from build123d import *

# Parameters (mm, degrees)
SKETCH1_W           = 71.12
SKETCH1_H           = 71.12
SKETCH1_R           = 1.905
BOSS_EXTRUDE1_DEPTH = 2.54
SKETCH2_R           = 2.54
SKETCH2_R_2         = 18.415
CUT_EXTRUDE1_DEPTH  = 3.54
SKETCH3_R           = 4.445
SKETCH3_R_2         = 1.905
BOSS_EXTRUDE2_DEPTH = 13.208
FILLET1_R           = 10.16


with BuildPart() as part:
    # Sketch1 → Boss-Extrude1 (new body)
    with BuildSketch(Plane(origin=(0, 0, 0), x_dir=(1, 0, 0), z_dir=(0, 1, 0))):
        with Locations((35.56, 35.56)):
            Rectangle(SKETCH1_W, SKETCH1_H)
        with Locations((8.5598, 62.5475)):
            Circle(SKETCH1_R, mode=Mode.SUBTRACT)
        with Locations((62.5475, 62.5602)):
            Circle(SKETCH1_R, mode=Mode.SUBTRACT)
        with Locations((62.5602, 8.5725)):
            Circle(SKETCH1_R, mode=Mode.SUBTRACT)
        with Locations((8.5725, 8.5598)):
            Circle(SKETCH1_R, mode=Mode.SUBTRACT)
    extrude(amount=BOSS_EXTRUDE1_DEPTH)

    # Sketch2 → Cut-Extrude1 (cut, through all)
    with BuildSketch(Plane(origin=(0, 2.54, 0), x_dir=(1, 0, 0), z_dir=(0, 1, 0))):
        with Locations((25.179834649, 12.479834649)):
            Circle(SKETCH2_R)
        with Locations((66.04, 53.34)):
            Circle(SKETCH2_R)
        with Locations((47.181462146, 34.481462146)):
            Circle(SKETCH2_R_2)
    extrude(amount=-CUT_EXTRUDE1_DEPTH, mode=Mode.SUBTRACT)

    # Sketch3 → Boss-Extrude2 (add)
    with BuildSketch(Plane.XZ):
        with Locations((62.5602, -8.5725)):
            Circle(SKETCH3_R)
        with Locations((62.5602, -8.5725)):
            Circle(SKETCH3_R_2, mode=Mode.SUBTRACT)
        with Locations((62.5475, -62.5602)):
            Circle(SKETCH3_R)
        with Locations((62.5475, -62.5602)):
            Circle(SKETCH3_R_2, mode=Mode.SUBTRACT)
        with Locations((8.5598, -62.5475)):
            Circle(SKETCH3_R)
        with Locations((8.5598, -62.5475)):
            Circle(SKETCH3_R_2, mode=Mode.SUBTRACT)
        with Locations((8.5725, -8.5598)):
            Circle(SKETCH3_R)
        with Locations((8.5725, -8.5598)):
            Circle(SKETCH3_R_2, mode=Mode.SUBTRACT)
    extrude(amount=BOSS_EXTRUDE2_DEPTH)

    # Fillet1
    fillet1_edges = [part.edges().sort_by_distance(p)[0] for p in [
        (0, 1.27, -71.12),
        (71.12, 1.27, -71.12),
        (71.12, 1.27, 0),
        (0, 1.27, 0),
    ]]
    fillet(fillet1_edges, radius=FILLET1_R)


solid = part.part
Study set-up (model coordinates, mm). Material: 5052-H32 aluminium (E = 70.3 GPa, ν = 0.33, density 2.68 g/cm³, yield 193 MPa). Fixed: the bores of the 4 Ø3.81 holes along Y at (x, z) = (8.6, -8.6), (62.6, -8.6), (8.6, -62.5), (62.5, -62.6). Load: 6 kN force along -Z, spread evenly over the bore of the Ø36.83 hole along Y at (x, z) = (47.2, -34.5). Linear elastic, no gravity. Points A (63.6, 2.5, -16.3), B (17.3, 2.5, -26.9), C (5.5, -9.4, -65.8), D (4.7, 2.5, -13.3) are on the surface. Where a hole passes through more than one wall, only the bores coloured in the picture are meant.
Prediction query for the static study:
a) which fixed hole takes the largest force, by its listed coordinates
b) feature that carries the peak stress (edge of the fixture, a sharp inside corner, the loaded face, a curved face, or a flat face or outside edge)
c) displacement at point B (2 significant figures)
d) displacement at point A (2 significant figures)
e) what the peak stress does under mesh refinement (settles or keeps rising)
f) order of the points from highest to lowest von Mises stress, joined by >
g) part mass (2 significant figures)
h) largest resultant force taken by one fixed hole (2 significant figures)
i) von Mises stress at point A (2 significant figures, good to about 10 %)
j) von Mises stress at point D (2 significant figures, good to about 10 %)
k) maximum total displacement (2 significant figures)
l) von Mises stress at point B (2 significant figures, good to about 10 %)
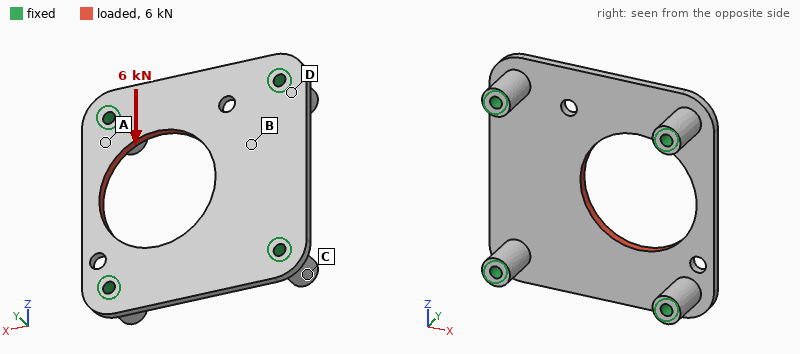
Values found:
(62.6, -8.6)
edge of the fixture
8.6 µm
5.7 µm
keeps rising
A > B > D > C
33 g
1.9 kN
45 MPa
15 MPa
23 µm
25 MPa
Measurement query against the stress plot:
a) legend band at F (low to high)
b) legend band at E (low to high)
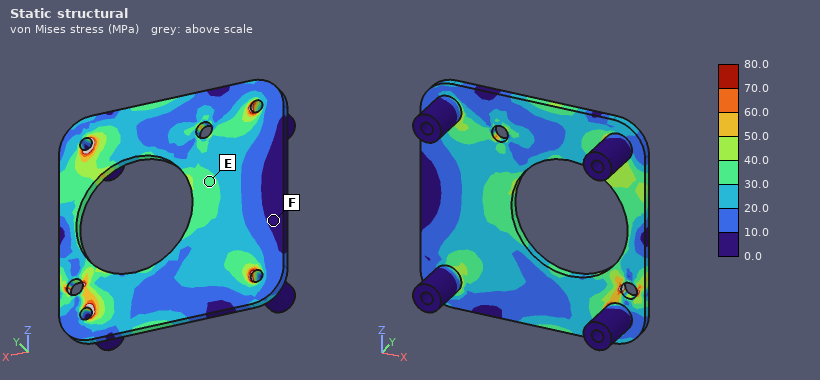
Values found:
0.0 to 10.0 MPa
30.0 to 40.0 MPa
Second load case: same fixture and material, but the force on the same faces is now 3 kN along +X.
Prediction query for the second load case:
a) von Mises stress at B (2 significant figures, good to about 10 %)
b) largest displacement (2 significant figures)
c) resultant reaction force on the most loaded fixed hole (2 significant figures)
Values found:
6.7 MPa
32 µm
930 N
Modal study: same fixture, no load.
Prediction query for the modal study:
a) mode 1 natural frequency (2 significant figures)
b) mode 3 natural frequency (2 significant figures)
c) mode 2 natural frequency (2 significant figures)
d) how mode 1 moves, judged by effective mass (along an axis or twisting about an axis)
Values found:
4100 Hz
5700 Hz
5600 Hz
along Y
